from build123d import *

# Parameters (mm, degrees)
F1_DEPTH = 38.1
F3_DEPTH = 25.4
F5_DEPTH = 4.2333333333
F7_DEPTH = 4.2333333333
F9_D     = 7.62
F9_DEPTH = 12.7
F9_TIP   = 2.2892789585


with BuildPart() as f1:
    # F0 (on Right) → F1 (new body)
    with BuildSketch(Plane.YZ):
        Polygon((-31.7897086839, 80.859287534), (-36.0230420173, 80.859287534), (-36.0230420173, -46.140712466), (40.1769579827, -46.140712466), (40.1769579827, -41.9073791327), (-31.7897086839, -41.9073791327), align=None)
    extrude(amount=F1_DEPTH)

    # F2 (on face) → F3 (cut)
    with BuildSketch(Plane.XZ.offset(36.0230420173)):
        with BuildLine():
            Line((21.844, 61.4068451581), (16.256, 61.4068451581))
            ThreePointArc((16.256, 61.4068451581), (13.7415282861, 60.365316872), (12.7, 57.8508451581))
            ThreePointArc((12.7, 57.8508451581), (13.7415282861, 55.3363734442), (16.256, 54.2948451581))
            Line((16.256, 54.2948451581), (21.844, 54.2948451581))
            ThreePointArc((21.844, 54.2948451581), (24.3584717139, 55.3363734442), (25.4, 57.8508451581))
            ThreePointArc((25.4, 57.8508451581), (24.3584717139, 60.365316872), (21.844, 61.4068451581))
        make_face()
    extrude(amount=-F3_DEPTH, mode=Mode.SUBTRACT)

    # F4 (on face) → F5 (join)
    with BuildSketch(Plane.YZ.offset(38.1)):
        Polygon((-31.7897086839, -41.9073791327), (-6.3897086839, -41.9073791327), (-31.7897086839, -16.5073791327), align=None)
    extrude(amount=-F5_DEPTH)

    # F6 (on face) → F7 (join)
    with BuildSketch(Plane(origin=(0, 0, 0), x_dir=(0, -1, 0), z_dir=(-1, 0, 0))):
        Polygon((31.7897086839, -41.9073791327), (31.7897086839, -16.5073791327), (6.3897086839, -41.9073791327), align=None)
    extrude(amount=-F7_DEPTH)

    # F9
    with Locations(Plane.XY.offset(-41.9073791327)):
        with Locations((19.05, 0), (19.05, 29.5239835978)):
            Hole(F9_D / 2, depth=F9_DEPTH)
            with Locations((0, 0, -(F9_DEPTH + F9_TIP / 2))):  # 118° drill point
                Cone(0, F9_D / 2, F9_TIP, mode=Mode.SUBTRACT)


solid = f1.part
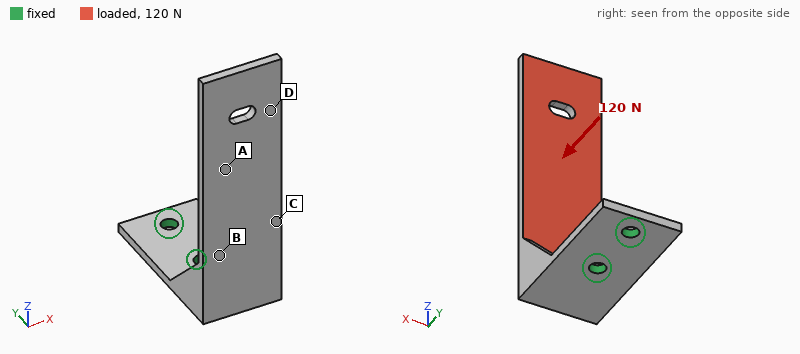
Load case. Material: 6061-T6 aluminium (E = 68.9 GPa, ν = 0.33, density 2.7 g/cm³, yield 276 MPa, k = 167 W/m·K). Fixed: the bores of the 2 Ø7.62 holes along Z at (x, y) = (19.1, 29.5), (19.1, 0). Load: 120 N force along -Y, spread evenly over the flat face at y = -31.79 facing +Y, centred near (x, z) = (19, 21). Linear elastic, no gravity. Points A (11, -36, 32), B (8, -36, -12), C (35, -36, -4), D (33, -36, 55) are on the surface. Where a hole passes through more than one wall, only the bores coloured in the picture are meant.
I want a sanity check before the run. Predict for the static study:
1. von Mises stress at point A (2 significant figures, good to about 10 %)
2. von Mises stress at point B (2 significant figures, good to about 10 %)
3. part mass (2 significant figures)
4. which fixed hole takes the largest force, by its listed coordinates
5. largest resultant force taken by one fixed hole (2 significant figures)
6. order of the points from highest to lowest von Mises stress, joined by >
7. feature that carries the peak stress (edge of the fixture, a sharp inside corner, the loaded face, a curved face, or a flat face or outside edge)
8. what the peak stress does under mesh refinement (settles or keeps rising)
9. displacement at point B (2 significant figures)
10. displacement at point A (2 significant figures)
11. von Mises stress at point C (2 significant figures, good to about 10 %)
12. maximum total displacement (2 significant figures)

11 MPa
40 MPa
92 g
(19.1, 29.5)
95 N
B > C > A > D
edge of the fixture
keeps rising
0.27 mm
0.83 mm
33 MPa
1.7 mm
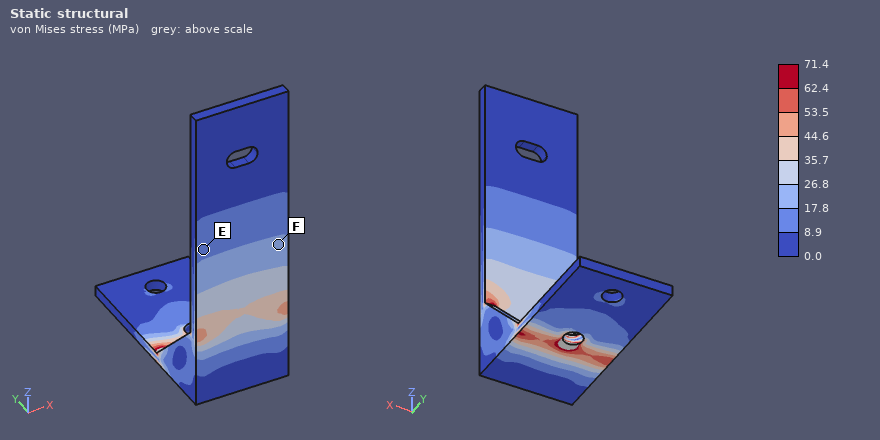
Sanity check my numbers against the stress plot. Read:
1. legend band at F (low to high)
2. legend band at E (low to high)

17.8 to 26.8 MPa
8.9 to 17.8 MPa
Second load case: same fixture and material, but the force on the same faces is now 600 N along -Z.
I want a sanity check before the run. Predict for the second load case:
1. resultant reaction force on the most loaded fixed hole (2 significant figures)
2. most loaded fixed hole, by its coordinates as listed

740 N
(19.1, 0)
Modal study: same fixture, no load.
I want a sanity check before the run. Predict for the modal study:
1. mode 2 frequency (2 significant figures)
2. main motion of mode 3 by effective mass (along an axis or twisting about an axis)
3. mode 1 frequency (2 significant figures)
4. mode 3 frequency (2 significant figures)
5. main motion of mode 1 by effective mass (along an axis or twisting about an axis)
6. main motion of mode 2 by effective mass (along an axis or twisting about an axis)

380 Hz
along Z
240 Hz
930 Hz
along Y
along X
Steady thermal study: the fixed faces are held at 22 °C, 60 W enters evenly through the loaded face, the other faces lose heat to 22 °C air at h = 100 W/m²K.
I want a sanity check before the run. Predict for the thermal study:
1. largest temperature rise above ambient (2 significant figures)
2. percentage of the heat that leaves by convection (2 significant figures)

69 K
66 %
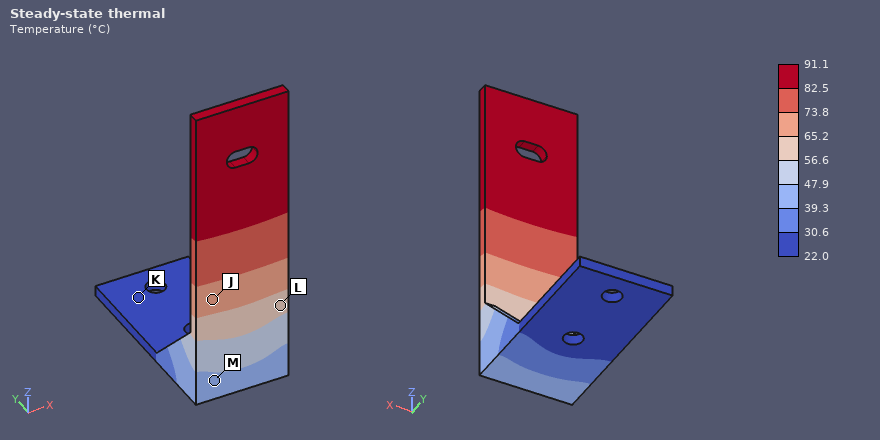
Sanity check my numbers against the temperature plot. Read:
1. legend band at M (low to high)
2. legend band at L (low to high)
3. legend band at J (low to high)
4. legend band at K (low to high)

39.3 to 47.9 °C
56.6 to 65.2 °C
65.2 to 73.8 °C
22.0 to 30.6 °C
